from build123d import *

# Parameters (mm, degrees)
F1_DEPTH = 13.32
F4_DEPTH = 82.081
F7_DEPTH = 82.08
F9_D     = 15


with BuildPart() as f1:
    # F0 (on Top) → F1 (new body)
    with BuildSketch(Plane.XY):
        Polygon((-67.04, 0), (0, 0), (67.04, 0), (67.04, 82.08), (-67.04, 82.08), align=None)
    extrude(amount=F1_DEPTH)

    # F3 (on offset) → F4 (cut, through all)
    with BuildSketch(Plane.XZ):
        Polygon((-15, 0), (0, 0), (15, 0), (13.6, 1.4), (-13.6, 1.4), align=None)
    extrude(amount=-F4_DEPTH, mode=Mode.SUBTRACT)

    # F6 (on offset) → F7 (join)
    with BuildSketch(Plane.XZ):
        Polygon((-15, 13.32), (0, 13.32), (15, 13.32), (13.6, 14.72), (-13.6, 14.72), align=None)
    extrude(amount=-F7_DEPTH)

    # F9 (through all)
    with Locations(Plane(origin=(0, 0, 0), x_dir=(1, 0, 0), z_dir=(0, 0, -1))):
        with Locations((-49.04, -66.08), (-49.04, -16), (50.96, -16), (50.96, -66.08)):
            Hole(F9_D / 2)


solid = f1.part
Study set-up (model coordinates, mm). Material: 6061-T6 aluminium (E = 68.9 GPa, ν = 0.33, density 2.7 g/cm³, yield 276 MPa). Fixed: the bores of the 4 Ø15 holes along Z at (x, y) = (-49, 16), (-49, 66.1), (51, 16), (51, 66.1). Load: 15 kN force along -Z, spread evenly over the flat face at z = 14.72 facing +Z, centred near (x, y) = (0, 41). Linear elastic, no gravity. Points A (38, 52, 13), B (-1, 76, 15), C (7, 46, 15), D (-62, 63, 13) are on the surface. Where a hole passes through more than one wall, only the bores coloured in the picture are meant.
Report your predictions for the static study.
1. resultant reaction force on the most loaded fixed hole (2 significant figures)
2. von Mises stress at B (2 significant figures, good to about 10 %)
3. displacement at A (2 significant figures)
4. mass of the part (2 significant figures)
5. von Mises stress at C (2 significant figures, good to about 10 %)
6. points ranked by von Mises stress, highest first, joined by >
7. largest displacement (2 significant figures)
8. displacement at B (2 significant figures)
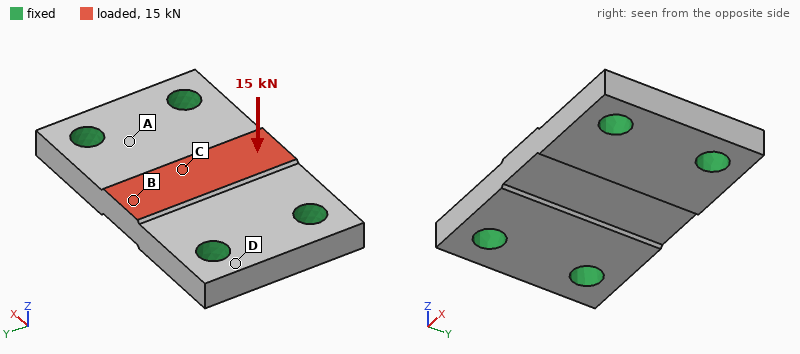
4.2 kN
51 MPa
13 µm
370 g
37 MPa
B > C > A > D
66 µm
63 µm
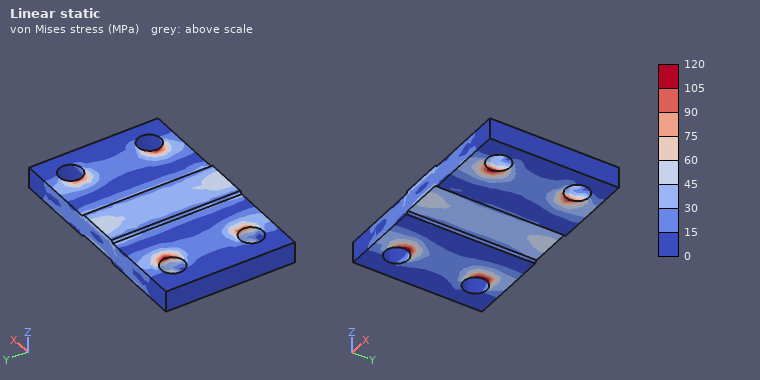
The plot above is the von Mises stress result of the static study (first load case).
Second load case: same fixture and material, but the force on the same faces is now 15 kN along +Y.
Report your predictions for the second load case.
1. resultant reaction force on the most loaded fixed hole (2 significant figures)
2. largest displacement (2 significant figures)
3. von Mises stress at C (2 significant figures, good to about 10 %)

4.9 kN
36 µm
16 MPa
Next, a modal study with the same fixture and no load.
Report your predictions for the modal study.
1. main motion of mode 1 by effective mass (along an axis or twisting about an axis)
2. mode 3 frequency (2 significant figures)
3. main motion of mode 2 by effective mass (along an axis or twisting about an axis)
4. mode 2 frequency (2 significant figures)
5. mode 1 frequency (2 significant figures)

along Z
14 kHz
twisting about X
8800 Hz
7200 Hz
